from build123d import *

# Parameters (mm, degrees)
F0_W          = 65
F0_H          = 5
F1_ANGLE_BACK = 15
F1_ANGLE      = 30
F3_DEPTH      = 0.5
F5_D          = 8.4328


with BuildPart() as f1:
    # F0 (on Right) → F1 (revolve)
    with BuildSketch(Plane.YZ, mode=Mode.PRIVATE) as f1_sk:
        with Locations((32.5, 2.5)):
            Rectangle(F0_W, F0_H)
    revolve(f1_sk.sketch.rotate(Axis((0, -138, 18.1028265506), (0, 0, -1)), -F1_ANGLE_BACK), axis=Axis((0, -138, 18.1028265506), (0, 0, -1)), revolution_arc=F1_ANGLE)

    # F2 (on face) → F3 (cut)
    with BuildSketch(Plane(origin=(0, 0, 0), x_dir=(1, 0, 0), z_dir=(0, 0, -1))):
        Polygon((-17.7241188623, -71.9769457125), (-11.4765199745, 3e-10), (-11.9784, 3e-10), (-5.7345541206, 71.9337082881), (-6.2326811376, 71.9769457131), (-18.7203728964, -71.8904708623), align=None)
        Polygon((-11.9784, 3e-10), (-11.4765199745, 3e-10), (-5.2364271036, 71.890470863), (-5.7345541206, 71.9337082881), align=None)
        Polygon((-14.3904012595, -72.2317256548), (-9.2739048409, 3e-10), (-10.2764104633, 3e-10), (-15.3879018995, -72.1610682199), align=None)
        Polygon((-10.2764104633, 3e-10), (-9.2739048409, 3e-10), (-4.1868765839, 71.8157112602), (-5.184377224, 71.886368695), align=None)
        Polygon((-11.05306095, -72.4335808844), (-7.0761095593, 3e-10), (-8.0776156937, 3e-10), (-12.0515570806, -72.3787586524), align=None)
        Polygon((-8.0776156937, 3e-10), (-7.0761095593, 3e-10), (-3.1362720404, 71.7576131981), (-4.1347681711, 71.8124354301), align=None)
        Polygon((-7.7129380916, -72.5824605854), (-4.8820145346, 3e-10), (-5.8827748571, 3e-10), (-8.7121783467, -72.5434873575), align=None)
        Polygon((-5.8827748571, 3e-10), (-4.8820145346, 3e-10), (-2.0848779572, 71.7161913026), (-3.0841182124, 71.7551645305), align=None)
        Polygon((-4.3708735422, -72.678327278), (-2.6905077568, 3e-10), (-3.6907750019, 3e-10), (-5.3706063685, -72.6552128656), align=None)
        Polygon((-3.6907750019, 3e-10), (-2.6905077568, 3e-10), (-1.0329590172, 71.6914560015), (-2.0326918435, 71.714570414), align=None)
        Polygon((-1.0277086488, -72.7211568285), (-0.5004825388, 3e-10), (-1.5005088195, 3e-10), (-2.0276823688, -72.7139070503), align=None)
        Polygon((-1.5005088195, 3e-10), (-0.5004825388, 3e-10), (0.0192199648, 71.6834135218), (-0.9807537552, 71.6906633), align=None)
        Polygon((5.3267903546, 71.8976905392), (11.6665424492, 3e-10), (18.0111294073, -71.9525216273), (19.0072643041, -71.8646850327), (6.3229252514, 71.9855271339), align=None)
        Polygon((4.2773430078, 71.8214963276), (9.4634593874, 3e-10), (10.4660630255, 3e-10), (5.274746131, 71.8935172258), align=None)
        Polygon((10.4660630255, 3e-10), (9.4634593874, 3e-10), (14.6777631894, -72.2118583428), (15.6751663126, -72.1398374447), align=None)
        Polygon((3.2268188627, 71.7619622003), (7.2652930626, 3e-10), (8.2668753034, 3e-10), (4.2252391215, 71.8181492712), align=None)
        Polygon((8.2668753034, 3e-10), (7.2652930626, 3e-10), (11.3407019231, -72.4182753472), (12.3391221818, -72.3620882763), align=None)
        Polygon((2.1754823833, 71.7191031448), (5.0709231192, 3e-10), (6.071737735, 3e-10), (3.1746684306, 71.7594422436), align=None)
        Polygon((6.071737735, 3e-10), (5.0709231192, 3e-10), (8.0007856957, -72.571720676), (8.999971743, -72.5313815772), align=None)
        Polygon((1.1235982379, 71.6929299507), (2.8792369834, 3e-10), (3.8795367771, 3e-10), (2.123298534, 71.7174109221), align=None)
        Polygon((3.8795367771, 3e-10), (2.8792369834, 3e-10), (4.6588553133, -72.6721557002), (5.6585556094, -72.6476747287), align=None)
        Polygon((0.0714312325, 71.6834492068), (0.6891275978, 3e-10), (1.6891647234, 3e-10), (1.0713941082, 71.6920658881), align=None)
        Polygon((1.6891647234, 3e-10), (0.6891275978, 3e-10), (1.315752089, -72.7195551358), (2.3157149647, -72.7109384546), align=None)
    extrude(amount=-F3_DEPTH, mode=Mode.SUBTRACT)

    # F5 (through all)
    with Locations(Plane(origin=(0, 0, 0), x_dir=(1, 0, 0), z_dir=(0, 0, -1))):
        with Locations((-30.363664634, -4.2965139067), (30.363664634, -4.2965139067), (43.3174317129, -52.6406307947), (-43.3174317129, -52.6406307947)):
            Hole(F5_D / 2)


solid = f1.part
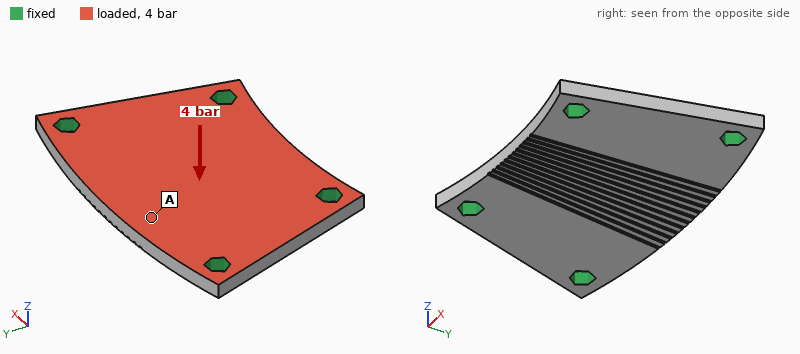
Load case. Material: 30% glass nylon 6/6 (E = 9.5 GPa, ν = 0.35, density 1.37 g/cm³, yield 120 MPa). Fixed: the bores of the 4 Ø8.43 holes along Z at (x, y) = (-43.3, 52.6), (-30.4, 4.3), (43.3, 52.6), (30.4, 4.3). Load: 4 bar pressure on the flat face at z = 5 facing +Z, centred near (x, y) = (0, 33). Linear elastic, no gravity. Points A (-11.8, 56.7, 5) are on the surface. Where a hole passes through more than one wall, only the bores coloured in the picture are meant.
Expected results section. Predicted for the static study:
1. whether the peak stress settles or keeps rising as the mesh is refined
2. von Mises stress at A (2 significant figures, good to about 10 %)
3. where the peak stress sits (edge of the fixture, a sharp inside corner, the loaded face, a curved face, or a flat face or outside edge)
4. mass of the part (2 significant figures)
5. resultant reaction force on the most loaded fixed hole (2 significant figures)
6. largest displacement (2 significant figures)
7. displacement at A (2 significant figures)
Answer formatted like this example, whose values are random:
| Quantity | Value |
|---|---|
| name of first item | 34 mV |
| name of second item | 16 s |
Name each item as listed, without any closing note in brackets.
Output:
| Quantity | Value |
|---|---|
| whether the peak stress settles or keeps rising as the mesh is refined | keeps rising |
| von Mises stress at A | 22 MPa |
| where the peak stress sits | edge of the fixture |
| mass of the part | 38 g |
| resultant reaction force on the most loaded fixed hole | 600 N |
| largest displacement | 0.63 mm |
| displacement at A | 0.47 mm |
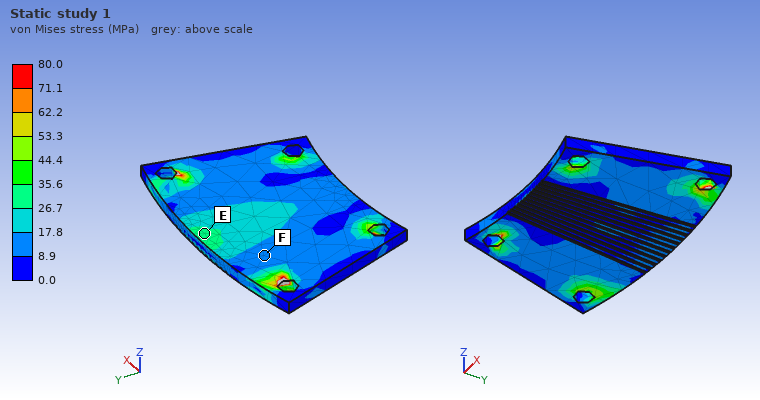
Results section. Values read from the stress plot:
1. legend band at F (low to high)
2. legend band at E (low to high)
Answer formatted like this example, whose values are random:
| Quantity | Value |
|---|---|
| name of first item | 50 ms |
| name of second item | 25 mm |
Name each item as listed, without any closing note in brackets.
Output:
| Quantity | Value |
|---|---|
| legend band at F | 8.9 to 17.8 MPa |
| legend band at E | 26.7 to 35.6 MPa |
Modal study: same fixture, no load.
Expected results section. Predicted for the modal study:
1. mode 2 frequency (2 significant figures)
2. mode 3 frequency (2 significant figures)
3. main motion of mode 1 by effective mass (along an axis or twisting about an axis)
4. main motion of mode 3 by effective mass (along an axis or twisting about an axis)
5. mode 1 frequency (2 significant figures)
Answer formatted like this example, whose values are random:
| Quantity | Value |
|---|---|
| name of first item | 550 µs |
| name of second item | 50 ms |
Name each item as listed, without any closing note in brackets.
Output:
| Quantity | Value |
|---|---|
| mode 2 frequency | 3700 Hz |
| mode 3 frequency | 5100 Hz |
| main motion of mode 1 by effective mass | along Z |
| main motion of mode 3 by effective mass | twisting about Y |
| mode 1 frequency | 2000 Hz |
